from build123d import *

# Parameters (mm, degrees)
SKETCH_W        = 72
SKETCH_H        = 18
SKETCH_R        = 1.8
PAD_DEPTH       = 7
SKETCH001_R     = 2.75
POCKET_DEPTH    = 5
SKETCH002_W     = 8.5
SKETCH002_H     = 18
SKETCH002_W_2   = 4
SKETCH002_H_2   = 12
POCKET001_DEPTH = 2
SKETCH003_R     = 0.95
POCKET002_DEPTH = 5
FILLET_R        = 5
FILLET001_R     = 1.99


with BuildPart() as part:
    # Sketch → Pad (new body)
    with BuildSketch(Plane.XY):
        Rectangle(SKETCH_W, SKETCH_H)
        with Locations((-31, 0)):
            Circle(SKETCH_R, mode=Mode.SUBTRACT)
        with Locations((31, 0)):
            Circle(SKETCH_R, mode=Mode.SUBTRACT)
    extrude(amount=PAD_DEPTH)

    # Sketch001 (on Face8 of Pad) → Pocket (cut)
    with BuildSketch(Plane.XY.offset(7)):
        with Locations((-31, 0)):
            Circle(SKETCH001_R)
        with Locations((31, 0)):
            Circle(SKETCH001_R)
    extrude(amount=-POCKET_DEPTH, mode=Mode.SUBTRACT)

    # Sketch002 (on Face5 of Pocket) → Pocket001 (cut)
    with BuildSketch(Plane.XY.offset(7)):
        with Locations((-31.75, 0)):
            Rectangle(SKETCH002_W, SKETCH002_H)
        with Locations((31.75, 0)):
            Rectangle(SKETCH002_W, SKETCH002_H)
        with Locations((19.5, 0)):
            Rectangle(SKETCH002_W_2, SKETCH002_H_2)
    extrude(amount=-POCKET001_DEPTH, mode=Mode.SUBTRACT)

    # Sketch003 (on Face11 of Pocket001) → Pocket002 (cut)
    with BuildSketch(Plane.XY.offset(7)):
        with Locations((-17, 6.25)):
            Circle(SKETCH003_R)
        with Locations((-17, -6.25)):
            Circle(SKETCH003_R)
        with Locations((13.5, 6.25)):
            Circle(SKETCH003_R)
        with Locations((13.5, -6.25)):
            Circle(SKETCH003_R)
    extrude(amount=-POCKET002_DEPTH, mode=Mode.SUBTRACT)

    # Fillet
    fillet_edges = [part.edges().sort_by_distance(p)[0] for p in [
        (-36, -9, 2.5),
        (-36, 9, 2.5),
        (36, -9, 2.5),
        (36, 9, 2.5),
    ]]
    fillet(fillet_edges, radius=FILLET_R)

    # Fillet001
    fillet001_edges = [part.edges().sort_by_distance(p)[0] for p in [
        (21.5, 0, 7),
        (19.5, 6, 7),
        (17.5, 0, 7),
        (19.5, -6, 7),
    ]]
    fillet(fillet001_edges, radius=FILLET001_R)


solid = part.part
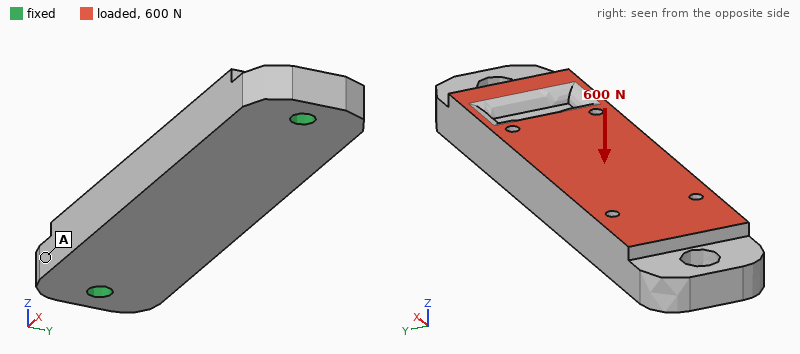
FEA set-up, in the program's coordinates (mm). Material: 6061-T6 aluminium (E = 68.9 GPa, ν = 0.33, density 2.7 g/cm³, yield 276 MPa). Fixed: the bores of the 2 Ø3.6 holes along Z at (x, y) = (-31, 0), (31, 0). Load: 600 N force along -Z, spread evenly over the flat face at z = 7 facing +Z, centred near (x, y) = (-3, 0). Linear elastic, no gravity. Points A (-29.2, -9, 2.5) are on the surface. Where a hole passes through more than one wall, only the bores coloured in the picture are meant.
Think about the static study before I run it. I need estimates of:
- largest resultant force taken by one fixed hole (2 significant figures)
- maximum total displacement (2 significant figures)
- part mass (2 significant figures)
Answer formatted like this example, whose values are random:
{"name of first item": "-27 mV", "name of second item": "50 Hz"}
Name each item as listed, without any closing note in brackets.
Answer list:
{"largest resultant force taken by one fixed hole": "600 N", "maximum total displacement": "31 µm", "part mass": "22 g"}
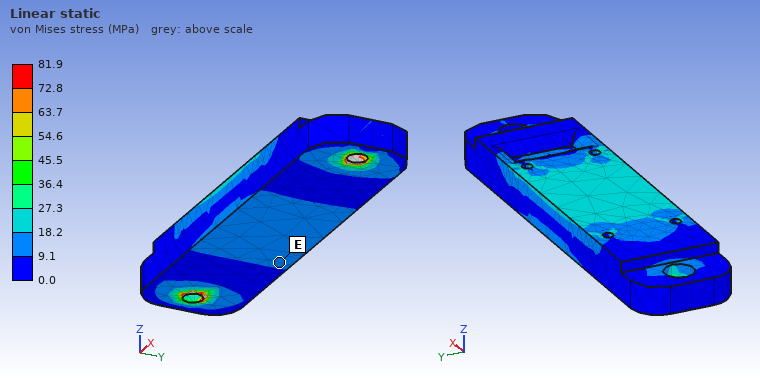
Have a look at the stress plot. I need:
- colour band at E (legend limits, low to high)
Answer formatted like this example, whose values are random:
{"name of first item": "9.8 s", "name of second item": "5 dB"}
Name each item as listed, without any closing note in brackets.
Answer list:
{"colour band at E": "9.1 to 18.2 MPa"}
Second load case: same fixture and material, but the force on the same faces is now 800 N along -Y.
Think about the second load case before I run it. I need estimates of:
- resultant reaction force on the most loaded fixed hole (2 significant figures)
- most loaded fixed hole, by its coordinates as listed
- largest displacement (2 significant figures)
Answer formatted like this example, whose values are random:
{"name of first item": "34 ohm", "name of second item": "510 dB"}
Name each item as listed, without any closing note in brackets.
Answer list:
{"resultant reaction force on the most loaded fixed hole": "440 N", "most loaded fixed hole, by its coordinates as listed": "(-31, 0)", "largest displacement": "41 µm"}
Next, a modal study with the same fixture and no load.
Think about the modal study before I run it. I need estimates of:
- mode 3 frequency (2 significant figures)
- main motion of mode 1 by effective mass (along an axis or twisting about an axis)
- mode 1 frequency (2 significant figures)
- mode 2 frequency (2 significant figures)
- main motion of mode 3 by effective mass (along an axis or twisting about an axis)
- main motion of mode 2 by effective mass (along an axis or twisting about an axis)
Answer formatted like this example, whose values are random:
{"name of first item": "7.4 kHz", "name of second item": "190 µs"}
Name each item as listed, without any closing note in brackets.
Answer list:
{"mode 3 frequency": "11 kHz", "main motion of mode 1 by effective mass": "along Z", "mode 1 frequency": "6000 Hz", "mode 2 frequency": "7200 Hz", "main motion of mode 3 by effective mass": "along Y", "main motion of mode 2 by effective mass": "along Y"}
